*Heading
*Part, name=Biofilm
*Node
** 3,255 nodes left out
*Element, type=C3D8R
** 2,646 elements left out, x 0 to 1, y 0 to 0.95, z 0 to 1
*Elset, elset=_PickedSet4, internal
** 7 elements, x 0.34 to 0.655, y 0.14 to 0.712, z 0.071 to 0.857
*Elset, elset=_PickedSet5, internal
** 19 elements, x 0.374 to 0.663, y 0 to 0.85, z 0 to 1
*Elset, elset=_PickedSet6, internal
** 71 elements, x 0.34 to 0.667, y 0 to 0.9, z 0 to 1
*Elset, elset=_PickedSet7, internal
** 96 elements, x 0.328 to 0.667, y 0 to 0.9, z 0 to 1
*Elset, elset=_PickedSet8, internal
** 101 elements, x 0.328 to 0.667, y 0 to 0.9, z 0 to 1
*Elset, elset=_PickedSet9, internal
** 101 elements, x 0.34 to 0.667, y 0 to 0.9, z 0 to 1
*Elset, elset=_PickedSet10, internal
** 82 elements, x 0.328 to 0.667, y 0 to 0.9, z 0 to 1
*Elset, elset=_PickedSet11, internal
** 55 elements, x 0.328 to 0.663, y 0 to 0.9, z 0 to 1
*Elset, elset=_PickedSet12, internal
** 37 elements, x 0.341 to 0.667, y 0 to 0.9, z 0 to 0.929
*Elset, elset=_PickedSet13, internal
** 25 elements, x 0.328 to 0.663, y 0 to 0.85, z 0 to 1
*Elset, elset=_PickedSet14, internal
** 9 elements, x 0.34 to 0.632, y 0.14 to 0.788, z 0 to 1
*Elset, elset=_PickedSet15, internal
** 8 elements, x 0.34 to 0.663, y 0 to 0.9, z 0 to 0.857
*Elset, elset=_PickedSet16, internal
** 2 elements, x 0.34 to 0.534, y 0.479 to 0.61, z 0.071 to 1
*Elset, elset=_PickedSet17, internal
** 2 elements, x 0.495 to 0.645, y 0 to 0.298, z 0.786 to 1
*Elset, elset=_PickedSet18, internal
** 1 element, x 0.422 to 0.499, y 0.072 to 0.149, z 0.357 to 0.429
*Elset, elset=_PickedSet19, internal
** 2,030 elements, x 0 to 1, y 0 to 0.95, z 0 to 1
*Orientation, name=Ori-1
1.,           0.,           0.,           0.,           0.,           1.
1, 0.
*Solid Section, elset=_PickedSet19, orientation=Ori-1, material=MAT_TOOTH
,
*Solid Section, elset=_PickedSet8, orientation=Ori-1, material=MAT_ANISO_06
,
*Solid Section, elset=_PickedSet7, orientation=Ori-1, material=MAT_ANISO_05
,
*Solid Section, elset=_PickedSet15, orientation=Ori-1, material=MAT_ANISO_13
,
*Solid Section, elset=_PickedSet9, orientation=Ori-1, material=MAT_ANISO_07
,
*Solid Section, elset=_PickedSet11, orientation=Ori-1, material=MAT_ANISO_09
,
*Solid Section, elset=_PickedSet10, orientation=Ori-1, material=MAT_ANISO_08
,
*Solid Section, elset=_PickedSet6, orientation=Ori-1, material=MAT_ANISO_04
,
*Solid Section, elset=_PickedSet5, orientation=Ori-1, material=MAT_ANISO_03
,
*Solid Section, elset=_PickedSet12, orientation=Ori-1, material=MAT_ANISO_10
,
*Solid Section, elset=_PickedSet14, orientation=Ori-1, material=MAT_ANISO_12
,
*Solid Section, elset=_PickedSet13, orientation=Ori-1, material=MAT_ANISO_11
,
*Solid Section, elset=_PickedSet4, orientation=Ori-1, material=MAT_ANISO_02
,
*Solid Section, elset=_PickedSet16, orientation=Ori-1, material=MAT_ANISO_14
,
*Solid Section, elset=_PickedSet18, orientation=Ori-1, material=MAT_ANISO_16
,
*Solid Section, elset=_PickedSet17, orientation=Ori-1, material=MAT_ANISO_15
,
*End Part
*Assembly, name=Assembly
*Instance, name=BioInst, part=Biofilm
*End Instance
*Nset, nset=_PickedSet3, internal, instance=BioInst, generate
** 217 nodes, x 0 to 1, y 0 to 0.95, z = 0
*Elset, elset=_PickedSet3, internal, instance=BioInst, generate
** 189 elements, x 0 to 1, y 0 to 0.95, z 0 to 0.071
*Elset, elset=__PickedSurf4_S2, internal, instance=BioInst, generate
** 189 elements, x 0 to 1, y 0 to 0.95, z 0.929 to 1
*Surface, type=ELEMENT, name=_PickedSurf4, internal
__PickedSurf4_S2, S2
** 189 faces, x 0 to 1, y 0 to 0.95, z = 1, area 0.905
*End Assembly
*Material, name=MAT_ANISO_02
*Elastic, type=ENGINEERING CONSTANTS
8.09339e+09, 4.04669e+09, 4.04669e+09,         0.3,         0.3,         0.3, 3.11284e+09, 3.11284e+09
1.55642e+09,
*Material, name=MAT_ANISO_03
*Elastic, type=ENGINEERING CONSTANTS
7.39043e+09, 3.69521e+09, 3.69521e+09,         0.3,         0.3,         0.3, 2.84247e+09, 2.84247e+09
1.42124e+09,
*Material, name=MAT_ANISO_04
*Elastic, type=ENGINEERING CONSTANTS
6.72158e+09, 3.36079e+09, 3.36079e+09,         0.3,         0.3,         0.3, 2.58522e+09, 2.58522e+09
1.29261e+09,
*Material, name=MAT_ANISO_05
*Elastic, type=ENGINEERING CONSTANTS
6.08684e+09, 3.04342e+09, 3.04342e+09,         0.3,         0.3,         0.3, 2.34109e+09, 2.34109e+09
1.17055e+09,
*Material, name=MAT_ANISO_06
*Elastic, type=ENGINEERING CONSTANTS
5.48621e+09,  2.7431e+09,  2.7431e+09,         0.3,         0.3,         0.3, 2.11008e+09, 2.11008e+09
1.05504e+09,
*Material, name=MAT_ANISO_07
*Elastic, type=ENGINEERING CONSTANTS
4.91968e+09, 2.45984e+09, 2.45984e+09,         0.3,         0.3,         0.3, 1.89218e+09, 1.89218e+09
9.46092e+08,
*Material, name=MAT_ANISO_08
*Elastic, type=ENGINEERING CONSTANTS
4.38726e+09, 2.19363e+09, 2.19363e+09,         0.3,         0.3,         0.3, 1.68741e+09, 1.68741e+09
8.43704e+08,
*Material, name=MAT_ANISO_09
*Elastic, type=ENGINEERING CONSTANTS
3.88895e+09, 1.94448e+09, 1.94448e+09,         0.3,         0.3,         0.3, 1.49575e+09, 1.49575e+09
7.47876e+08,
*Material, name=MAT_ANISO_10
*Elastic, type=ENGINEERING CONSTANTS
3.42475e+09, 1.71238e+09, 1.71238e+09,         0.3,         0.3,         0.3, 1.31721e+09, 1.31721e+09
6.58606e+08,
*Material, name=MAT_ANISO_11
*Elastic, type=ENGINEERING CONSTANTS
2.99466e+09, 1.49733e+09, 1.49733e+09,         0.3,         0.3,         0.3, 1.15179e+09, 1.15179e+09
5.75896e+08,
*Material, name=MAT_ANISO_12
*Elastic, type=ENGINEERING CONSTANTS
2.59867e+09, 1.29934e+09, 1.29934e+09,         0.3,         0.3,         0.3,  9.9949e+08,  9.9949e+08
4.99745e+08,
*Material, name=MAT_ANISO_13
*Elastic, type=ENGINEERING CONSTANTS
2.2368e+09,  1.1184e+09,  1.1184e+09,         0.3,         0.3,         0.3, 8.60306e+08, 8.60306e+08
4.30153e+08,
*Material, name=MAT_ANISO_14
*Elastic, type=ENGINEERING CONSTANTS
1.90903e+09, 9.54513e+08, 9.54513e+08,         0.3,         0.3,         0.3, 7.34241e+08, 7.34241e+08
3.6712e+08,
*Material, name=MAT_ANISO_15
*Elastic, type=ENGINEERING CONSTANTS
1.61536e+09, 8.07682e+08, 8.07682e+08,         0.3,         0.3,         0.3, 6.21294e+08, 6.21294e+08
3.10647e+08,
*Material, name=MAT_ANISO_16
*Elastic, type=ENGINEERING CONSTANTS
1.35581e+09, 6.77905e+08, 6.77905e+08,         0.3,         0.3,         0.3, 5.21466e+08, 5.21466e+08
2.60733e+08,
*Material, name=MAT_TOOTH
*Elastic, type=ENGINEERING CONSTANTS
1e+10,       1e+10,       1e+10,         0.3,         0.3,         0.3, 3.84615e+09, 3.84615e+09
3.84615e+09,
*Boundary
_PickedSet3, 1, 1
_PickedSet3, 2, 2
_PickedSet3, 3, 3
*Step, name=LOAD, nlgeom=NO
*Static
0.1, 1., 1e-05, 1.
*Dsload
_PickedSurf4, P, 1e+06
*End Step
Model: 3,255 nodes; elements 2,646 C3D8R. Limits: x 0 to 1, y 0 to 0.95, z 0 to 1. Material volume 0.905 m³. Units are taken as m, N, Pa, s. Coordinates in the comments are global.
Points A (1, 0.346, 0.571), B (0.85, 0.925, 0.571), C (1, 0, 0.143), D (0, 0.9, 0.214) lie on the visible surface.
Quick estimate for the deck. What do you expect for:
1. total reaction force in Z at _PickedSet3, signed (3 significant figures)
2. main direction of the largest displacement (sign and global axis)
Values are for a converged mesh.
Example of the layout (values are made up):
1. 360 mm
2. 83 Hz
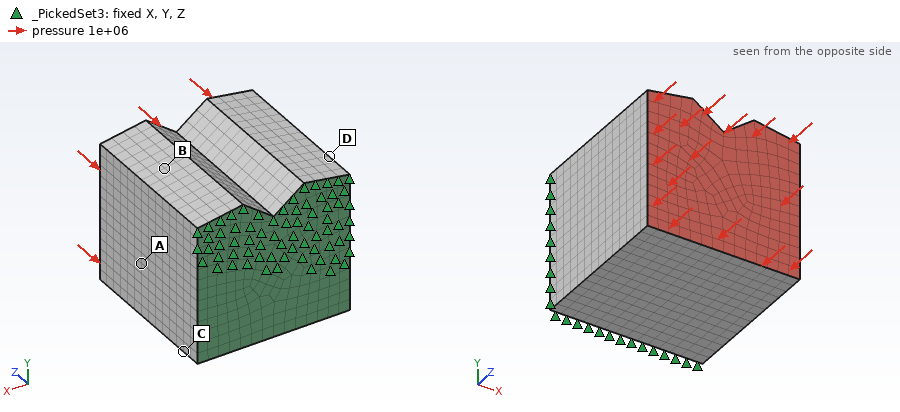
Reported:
1. 9.05e+05 N
2. -Z
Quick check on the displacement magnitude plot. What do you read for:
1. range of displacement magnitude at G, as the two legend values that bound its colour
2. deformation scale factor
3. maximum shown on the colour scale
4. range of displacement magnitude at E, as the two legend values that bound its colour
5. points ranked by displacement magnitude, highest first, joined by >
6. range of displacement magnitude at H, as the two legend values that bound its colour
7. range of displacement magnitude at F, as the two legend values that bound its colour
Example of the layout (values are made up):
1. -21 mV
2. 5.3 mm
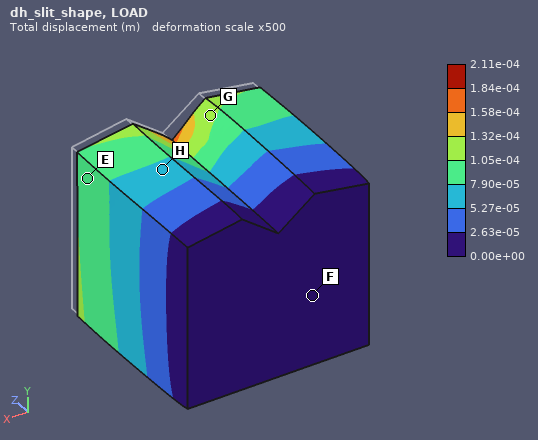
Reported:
1. 1.05e-04 to 1.32e-04 m
2. 500
3. 2.11e-04 m
4. 7.90e-05 to 1.05e-04 m
5. G > E > H > F
6. 5.27e-05 to 7.90e-05 m
7. 0.00e+00 to 2.63e-05 m
